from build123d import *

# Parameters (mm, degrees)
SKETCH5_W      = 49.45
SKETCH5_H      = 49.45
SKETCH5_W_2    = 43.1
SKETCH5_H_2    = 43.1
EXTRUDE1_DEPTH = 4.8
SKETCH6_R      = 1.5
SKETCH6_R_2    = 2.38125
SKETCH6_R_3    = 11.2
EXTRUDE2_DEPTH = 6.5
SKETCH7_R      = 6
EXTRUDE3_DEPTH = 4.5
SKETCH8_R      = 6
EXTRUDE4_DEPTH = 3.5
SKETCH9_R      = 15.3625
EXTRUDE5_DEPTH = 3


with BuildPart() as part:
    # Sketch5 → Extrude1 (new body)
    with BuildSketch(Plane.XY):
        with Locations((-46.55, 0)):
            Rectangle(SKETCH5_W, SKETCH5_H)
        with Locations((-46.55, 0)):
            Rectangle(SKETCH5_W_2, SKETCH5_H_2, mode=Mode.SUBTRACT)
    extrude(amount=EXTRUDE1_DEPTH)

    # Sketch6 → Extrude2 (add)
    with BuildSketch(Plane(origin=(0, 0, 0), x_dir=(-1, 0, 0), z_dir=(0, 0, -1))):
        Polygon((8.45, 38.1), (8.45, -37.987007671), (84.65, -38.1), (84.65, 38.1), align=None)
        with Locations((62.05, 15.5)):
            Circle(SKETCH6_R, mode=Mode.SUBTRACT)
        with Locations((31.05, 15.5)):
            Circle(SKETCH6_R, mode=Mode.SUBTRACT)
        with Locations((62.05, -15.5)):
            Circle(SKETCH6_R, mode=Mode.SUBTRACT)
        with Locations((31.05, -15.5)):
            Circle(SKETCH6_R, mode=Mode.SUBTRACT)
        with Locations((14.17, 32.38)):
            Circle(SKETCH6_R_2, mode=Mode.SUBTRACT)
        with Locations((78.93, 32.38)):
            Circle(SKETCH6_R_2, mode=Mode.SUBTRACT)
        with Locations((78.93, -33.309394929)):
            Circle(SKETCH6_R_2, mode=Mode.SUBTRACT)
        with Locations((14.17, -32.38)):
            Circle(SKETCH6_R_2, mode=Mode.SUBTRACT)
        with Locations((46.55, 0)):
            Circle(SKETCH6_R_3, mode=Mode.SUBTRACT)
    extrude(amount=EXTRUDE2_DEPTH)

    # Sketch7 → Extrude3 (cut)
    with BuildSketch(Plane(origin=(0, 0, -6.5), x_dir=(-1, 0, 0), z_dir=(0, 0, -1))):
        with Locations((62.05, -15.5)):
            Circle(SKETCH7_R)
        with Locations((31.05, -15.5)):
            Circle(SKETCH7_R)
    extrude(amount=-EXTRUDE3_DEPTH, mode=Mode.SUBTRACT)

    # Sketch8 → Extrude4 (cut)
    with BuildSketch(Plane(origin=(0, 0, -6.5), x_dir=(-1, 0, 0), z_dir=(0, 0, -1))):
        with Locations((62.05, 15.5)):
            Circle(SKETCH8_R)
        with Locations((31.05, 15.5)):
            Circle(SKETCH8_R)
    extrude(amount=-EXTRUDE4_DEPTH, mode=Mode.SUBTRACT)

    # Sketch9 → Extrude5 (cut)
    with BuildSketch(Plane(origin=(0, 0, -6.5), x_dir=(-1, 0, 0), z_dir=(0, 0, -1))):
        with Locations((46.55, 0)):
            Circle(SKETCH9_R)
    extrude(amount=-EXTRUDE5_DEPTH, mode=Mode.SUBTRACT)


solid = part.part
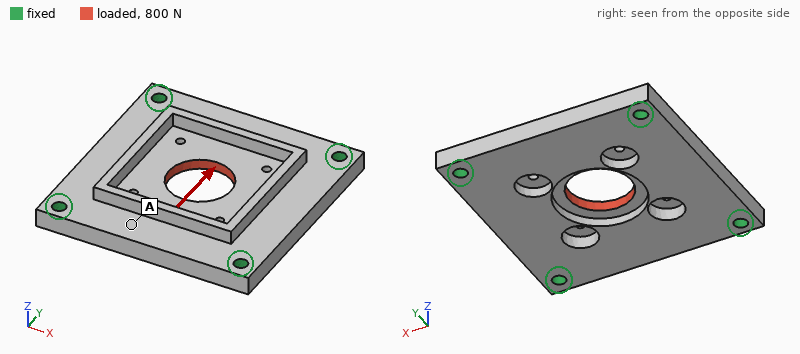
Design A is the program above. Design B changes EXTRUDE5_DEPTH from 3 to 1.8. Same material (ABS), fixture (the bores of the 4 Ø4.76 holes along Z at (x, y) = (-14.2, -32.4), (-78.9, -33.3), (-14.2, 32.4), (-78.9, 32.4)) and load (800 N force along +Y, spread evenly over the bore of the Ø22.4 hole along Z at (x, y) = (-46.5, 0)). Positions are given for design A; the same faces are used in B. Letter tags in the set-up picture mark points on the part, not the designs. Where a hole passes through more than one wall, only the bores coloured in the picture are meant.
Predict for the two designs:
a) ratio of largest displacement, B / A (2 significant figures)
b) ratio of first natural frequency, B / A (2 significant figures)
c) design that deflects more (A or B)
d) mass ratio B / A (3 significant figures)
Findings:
0.87
0.99
A
1.01
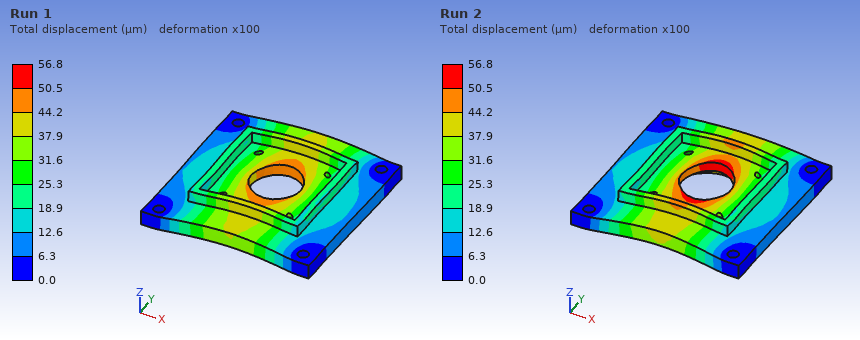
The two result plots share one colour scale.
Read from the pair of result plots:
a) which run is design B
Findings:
Run 1
